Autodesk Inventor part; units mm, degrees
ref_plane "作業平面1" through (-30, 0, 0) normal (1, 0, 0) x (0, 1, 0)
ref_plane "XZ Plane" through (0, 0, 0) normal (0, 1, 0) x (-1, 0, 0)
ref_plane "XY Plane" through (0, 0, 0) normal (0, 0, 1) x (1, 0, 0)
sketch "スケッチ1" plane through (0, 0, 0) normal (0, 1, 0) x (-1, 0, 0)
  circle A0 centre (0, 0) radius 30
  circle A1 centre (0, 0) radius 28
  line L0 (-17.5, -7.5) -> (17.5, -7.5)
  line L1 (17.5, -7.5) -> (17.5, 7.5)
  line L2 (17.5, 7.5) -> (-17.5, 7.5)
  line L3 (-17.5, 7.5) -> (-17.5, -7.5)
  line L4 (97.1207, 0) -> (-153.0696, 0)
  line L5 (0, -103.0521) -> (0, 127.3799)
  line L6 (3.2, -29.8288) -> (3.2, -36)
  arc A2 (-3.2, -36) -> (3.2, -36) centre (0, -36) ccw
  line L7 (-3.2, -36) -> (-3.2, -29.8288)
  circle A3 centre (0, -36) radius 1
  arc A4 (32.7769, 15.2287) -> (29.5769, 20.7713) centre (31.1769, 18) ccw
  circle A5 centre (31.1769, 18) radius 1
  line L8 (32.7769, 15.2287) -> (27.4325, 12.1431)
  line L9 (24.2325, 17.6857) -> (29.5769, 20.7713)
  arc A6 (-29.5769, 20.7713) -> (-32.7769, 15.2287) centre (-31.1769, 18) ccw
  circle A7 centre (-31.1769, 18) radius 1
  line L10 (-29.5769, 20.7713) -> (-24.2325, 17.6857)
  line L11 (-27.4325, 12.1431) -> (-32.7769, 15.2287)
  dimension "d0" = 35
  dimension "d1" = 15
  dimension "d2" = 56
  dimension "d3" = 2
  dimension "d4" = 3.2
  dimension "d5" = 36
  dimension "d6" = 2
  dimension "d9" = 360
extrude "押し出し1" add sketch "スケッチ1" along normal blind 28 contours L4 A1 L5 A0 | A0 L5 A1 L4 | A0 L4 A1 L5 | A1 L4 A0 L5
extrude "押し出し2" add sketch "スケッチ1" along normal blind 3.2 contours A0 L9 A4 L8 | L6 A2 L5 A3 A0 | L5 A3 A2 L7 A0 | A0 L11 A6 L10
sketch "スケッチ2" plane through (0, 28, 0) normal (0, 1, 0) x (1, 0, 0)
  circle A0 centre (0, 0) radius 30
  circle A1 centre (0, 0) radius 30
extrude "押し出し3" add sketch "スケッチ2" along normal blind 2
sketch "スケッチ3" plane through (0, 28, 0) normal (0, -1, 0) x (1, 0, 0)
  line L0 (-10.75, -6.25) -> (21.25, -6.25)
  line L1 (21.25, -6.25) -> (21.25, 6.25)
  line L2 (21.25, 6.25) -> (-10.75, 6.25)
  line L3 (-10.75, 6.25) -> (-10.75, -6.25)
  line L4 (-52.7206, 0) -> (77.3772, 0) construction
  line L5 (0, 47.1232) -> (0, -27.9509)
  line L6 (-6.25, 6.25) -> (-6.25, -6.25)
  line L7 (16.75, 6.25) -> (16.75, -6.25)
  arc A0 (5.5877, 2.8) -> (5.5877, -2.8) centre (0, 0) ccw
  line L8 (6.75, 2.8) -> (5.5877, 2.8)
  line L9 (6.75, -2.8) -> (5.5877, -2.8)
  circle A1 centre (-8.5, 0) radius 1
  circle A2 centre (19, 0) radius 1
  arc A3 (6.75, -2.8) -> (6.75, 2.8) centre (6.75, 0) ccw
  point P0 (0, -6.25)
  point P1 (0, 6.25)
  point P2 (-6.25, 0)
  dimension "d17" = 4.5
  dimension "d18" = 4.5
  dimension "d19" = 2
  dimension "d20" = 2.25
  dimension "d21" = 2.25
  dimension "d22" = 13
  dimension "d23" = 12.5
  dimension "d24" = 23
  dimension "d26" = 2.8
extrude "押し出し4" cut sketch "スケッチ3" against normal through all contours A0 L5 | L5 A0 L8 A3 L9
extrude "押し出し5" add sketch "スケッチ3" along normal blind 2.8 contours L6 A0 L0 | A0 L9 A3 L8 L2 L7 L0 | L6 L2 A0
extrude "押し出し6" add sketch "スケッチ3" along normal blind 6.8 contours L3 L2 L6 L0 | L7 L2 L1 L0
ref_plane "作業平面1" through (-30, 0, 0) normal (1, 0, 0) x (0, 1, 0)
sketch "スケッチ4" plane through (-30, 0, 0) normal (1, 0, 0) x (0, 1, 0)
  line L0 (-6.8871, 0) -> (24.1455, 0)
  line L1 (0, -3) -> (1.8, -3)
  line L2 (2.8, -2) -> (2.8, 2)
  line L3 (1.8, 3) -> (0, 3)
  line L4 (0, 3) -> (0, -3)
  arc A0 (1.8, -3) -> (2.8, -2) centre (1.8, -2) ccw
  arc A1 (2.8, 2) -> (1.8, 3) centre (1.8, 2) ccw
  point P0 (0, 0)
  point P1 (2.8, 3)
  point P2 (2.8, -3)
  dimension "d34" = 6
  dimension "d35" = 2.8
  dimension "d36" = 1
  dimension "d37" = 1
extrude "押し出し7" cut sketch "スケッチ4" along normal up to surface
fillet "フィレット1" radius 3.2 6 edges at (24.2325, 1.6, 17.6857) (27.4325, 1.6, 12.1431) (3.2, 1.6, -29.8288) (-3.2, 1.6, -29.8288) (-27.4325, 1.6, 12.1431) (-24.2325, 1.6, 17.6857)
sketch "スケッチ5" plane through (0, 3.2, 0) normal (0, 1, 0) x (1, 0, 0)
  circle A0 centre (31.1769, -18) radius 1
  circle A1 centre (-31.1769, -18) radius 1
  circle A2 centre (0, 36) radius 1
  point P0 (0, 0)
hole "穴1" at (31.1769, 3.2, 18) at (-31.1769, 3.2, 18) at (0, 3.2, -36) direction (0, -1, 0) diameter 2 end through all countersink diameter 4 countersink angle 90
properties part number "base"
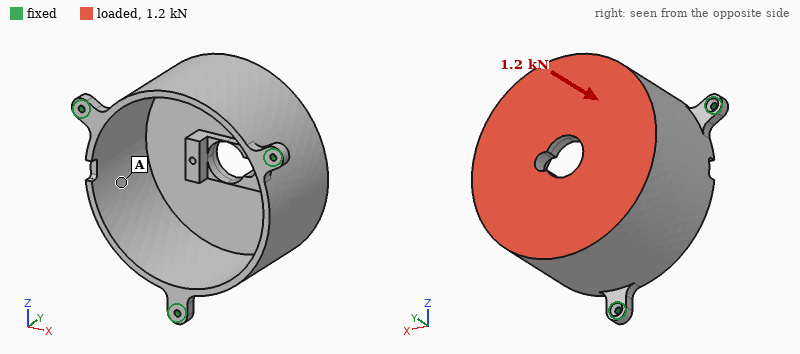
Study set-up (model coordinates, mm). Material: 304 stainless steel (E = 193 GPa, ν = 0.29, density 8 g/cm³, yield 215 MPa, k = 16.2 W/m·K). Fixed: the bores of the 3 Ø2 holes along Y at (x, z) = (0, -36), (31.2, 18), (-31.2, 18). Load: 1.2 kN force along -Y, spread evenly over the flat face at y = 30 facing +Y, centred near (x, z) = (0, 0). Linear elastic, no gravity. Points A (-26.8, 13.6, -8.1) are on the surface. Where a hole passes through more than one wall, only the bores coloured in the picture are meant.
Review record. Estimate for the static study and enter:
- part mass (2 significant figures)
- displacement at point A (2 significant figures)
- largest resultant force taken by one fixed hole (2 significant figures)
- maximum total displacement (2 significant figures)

140 g
12 µm
420 N
48 µm
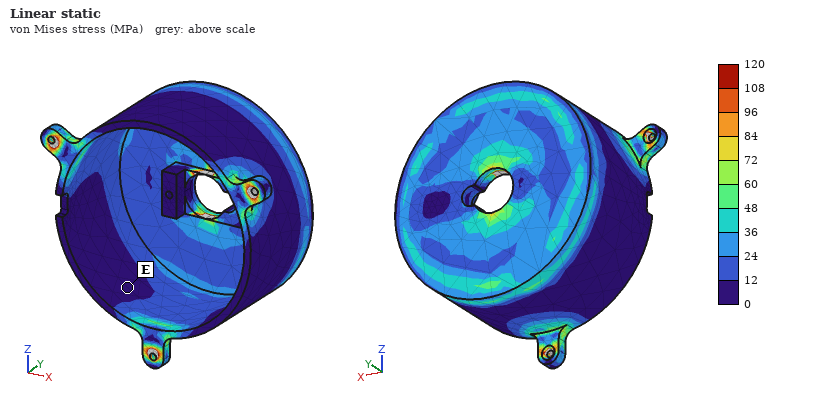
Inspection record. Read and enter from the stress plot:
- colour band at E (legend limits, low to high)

0 to 12 MPa
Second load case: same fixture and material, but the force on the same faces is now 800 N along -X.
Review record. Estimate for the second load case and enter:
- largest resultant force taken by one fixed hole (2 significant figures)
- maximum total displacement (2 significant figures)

490 N
21 µm
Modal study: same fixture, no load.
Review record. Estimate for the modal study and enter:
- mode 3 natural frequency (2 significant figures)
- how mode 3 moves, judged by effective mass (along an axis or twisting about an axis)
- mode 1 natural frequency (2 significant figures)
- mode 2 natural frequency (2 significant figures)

3700 Hz
along Y
3300 Hz
3400 Hz
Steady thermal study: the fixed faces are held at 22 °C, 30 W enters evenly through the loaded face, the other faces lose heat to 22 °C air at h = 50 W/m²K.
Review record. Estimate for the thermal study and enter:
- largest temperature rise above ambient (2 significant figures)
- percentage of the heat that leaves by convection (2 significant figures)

82 K
94 %
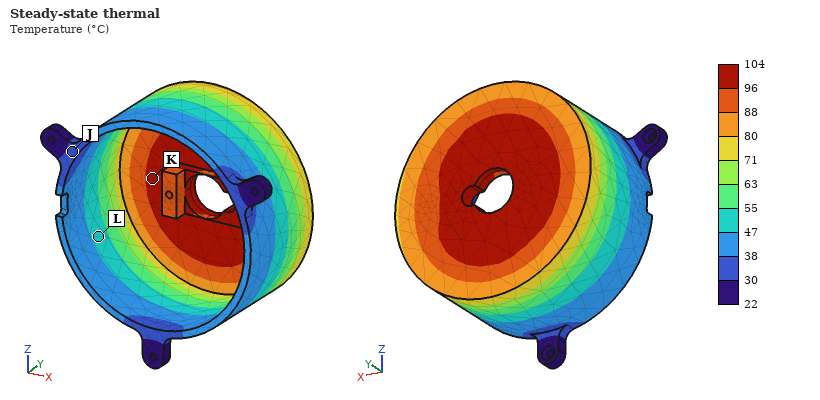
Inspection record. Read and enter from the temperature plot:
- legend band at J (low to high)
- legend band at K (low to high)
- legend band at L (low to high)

30 to 38 °C
96 to 104 °C
47 to 55 °C
